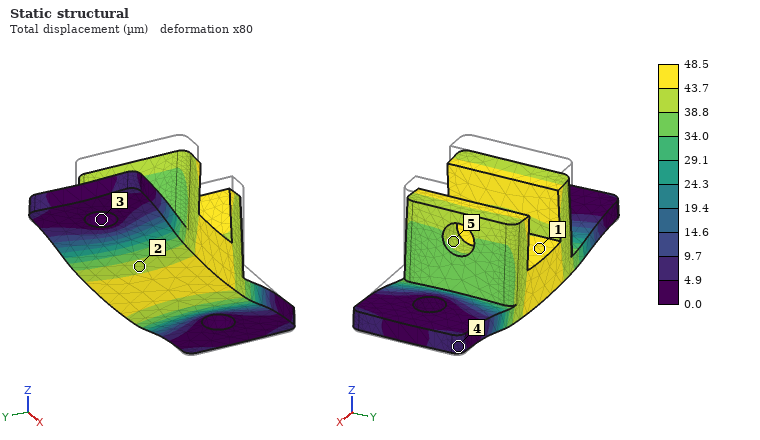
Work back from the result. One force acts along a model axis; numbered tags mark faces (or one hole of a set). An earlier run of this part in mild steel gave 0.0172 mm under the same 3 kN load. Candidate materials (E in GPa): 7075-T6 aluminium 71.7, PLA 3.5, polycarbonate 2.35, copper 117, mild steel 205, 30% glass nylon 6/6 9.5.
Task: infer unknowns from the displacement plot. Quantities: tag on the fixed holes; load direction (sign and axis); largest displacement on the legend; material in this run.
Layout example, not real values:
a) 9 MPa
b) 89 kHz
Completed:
a) 3
b) -Z
c) 48.5 µm
d) 7075-T6 aluminium
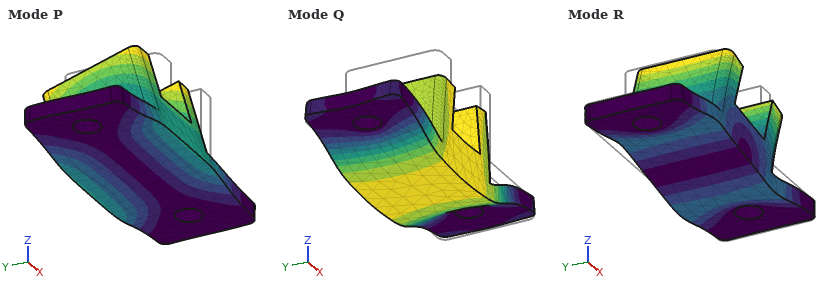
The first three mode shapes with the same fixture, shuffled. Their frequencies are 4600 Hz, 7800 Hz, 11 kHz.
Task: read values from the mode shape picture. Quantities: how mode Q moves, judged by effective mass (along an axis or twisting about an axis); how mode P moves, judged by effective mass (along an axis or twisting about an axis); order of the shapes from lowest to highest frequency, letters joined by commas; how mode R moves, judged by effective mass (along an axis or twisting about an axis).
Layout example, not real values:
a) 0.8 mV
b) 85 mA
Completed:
a) along Z
b) along Y
c) P, Q, R
d) along X
